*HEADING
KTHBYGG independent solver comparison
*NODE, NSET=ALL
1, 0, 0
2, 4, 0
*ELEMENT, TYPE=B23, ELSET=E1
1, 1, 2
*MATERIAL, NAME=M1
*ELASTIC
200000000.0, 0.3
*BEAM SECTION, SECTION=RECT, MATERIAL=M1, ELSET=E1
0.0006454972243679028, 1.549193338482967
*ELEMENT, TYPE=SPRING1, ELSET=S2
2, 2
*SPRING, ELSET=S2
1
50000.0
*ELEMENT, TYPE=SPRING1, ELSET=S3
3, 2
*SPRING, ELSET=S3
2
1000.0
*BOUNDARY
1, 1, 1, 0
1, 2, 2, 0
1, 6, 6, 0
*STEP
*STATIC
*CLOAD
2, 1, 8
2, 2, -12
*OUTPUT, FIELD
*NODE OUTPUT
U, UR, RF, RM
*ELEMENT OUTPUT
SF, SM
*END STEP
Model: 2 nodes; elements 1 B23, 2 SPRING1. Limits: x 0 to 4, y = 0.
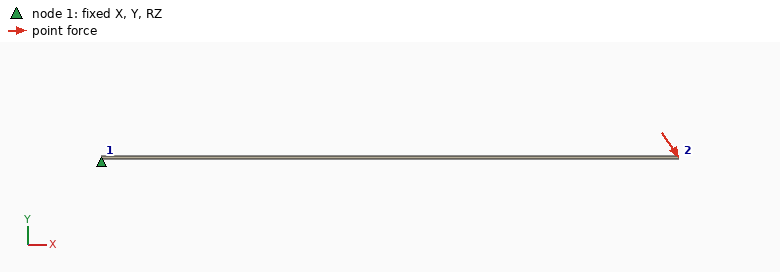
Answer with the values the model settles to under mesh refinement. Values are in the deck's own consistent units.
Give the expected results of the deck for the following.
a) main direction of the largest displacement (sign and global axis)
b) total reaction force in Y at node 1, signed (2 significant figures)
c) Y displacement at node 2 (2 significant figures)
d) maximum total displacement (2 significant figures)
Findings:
-Y
7.8
-0.0042
0.0042
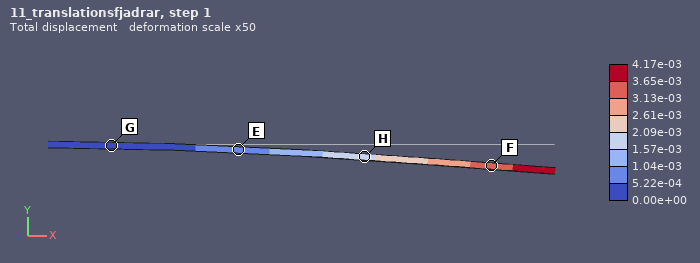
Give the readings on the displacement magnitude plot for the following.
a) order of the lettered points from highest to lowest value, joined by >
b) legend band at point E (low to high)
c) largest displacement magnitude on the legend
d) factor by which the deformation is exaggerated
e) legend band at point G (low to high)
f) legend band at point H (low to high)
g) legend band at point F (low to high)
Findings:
F > H > E > G
5.22e-04 to 1.04e-03
4.17e-03
50
0.00e+00 to 5.22e-04
1.57e-03 to 2.09e-03
3.13e-03 to 3.65e-03
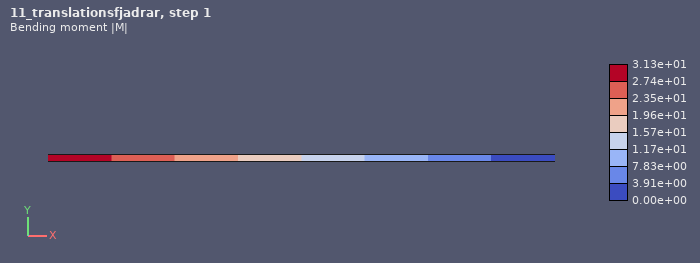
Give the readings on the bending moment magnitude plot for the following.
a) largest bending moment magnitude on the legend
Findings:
3.13e+01
